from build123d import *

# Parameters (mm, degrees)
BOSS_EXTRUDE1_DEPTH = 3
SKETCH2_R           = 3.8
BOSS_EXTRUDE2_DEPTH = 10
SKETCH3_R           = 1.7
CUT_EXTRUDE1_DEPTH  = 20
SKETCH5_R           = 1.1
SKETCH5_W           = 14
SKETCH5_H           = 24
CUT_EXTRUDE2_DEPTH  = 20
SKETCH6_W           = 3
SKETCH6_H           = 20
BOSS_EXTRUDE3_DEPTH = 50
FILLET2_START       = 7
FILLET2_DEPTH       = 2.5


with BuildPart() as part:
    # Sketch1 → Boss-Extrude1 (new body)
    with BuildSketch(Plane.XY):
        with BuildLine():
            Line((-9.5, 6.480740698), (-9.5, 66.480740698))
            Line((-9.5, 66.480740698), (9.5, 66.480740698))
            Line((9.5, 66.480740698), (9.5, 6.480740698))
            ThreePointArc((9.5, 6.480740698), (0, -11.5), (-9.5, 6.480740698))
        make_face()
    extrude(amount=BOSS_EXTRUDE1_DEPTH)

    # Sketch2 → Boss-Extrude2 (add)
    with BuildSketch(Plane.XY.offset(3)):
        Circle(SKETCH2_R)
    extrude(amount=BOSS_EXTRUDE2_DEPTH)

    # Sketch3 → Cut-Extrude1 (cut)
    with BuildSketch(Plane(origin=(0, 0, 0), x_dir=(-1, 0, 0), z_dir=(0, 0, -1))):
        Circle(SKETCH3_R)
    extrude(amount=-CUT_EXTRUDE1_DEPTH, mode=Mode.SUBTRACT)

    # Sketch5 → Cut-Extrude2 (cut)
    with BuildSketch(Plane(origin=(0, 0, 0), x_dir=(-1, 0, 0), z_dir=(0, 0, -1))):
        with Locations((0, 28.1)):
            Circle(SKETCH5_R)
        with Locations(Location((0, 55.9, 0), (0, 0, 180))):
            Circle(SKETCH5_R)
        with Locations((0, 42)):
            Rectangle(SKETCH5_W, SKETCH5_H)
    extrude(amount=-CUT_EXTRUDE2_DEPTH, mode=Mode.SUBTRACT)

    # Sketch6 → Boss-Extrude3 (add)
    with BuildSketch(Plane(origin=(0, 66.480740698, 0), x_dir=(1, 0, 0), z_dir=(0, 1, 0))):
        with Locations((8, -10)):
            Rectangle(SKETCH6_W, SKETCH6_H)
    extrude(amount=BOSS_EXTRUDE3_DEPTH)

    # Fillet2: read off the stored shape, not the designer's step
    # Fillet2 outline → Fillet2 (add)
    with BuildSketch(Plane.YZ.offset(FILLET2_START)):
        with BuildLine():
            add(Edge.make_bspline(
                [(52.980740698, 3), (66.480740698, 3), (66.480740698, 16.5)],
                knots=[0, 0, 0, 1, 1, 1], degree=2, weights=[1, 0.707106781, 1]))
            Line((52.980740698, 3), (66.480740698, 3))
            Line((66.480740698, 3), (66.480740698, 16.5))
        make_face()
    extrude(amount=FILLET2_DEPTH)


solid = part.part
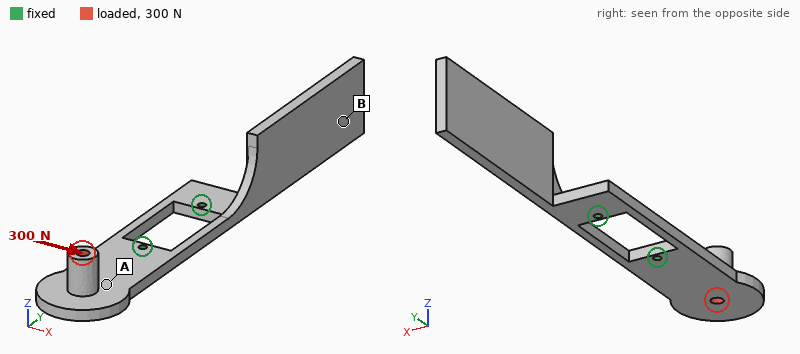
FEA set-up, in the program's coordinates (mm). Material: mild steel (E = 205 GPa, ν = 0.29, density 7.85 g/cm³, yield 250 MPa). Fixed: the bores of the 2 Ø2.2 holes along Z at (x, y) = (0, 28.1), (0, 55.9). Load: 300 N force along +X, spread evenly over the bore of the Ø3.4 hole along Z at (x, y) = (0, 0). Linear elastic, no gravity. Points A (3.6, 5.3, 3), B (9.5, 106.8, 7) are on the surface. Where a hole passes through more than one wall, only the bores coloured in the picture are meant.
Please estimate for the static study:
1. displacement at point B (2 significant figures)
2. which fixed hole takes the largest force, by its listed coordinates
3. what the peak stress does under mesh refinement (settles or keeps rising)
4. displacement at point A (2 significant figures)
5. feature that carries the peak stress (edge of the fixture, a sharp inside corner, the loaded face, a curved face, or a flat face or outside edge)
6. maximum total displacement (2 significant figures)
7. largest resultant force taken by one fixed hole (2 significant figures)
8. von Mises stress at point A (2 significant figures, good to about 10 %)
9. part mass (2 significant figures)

48 µm
(0, 28.1)
keeps rising
44 µm
edge of the fixture
96 µm
330 N
49 MPa
54 g
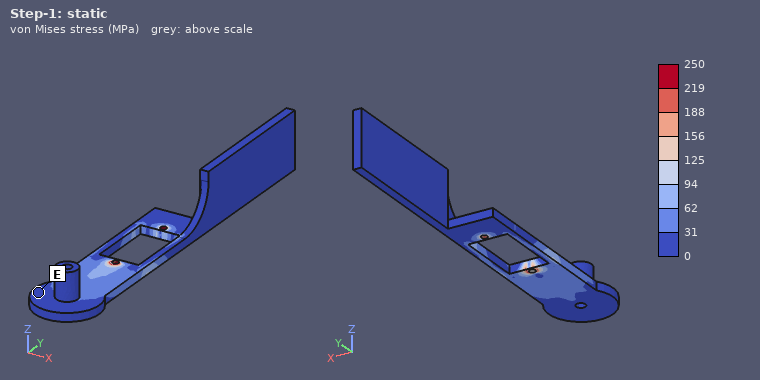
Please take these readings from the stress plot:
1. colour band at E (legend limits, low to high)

0 to 31 MPa
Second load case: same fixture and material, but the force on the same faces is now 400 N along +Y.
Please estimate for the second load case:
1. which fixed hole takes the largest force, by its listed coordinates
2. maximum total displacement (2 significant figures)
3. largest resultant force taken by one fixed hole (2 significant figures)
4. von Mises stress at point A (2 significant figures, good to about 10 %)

(0, 28.1)
0.18 mm
360 N
70 MPa
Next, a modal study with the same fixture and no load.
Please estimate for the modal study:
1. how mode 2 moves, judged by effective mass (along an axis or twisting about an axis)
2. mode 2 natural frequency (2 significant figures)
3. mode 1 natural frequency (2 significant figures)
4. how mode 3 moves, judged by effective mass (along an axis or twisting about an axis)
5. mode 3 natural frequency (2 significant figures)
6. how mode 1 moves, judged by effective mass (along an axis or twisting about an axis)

along Z
700 Hz
580 Hz
along Z
1300 Hz
along X
